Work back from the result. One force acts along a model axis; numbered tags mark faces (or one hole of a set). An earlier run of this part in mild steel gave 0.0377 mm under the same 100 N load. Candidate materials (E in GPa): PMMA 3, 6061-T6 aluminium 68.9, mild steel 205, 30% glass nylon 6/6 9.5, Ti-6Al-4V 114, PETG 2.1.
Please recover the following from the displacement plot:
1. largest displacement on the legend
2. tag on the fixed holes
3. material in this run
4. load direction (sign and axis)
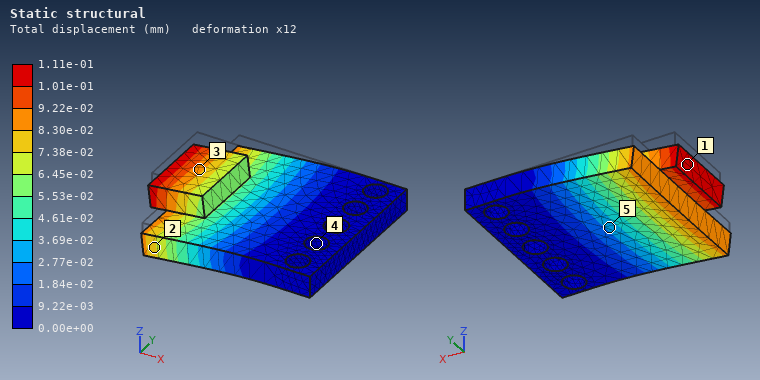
1.11e-01 mm
4
6061-T6 aluminium
-Z
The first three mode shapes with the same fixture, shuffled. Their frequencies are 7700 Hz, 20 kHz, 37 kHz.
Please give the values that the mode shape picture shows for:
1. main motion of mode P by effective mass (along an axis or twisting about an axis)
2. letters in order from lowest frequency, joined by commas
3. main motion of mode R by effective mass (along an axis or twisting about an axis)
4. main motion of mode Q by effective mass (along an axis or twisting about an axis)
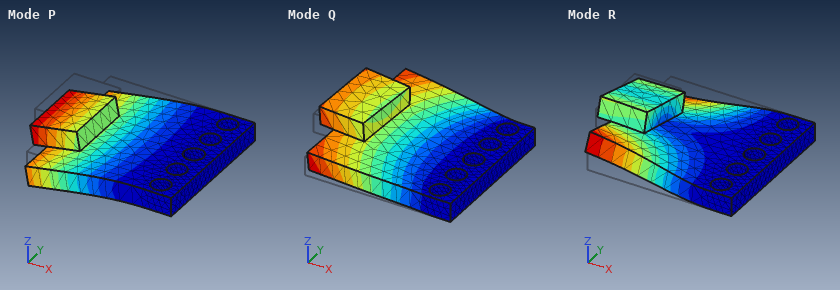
along Z
P, R, Q
twisting about X
along Y
